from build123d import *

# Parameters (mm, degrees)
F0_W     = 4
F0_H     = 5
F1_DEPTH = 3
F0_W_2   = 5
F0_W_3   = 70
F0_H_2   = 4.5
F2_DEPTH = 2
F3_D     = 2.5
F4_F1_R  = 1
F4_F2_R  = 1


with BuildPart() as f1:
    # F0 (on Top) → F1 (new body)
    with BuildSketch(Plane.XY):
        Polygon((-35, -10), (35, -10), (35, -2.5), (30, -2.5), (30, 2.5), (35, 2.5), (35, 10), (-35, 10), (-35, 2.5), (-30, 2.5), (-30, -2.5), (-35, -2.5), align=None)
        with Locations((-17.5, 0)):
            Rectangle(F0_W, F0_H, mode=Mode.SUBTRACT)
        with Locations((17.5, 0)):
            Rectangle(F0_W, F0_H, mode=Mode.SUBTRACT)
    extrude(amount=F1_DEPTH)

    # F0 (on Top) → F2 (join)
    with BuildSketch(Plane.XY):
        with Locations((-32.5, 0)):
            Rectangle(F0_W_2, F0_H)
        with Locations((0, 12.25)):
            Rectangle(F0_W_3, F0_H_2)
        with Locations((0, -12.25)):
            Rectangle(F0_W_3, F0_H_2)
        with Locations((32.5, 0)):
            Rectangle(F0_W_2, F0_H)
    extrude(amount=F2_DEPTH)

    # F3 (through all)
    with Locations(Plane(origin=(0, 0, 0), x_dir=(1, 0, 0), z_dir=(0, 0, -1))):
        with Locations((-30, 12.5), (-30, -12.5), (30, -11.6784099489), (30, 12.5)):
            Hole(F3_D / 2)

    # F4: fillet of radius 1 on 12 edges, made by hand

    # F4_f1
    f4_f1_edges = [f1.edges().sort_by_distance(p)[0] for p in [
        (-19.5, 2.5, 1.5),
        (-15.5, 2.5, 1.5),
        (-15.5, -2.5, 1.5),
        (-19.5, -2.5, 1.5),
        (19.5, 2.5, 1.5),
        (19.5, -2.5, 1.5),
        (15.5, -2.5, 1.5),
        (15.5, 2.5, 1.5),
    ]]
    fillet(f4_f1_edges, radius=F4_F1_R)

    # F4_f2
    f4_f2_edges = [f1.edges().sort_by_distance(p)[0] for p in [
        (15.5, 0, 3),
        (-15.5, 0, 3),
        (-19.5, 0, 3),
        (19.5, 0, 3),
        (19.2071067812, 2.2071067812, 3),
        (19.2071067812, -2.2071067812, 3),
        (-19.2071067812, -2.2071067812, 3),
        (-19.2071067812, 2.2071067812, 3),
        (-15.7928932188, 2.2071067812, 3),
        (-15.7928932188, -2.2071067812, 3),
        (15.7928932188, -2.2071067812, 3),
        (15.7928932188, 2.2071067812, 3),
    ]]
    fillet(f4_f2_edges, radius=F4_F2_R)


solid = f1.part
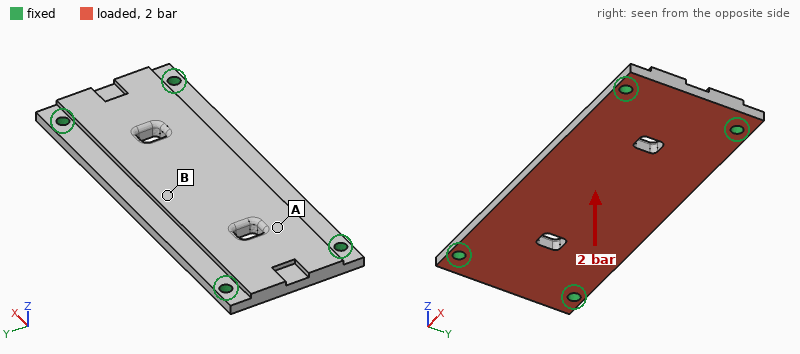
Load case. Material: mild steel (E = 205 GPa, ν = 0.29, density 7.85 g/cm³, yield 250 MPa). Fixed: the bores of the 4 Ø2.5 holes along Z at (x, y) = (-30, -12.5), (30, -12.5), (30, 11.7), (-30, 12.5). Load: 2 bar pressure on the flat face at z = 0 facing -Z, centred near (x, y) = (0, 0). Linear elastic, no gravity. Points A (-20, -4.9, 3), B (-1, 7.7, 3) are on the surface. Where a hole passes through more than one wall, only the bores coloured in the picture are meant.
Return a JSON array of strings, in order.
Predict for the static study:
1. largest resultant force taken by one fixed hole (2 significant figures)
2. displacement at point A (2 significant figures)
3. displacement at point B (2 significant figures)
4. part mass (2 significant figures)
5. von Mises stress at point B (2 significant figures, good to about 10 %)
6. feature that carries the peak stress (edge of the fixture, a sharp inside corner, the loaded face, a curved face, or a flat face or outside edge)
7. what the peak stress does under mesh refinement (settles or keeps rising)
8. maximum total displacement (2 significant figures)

["130 N", "12 µm", "28 µm", "41 g", "34 MPa", "edge of the fixture", "keeps rising", "30 µm"]
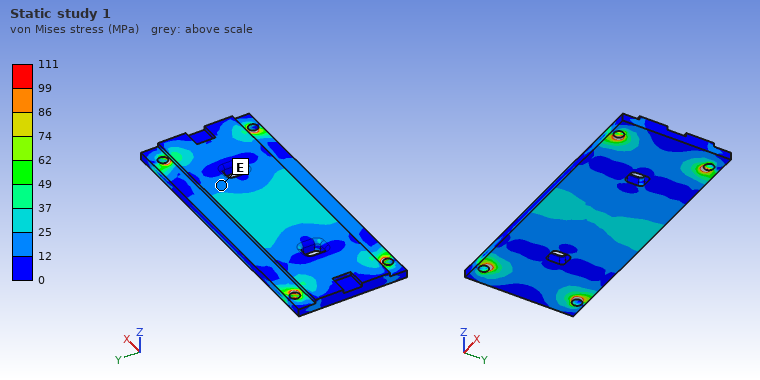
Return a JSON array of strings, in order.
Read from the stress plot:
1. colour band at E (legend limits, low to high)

["12 to 25 MPa"]
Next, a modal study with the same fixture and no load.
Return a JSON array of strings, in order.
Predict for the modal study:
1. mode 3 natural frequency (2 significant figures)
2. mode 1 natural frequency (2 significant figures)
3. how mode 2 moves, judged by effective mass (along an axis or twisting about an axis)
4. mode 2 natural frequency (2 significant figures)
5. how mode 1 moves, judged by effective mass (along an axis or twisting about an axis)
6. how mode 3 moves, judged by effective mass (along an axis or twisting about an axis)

["9000 Hz", "3300 Hz", "twisting about X", "6400 Hz", "along Z", "twisting about Y"]
